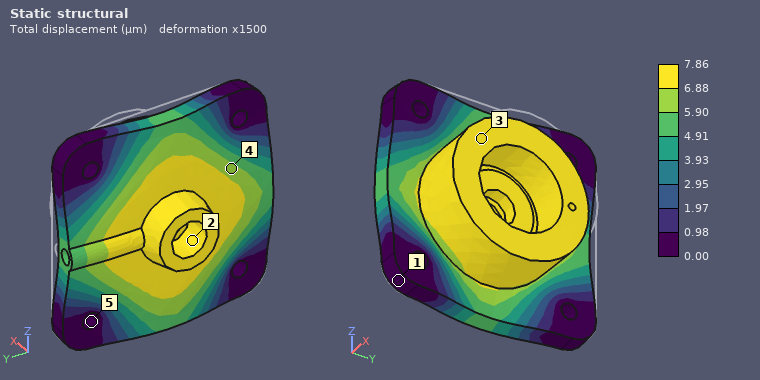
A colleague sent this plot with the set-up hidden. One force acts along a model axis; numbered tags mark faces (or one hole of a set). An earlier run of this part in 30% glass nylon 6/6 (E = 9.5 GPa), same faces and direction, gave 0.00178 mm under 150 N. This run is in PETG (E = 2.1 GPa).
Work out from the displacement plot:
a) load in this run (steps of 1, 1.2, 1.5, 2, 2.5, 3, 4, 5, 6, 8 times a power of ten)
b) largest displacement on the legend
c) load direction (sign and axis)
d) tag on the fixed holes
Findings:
150 N
7.86 µm
-X
5
